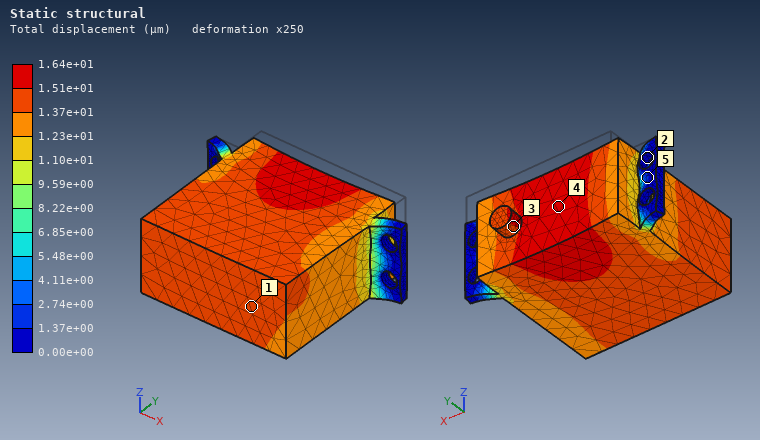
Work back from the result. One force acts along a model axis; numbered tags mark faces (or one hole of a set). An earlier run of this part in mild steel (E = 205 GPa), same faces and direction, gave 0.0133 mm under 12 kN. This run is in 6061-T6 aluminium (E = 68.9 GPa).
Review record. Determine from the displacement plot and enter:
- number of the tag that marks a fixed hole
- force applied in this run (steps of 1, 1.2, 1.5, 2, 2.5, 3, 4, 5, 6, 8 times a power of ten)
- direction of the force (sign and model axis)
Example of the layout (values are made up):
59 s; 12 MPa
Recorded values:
2; 5 kN; -Y
